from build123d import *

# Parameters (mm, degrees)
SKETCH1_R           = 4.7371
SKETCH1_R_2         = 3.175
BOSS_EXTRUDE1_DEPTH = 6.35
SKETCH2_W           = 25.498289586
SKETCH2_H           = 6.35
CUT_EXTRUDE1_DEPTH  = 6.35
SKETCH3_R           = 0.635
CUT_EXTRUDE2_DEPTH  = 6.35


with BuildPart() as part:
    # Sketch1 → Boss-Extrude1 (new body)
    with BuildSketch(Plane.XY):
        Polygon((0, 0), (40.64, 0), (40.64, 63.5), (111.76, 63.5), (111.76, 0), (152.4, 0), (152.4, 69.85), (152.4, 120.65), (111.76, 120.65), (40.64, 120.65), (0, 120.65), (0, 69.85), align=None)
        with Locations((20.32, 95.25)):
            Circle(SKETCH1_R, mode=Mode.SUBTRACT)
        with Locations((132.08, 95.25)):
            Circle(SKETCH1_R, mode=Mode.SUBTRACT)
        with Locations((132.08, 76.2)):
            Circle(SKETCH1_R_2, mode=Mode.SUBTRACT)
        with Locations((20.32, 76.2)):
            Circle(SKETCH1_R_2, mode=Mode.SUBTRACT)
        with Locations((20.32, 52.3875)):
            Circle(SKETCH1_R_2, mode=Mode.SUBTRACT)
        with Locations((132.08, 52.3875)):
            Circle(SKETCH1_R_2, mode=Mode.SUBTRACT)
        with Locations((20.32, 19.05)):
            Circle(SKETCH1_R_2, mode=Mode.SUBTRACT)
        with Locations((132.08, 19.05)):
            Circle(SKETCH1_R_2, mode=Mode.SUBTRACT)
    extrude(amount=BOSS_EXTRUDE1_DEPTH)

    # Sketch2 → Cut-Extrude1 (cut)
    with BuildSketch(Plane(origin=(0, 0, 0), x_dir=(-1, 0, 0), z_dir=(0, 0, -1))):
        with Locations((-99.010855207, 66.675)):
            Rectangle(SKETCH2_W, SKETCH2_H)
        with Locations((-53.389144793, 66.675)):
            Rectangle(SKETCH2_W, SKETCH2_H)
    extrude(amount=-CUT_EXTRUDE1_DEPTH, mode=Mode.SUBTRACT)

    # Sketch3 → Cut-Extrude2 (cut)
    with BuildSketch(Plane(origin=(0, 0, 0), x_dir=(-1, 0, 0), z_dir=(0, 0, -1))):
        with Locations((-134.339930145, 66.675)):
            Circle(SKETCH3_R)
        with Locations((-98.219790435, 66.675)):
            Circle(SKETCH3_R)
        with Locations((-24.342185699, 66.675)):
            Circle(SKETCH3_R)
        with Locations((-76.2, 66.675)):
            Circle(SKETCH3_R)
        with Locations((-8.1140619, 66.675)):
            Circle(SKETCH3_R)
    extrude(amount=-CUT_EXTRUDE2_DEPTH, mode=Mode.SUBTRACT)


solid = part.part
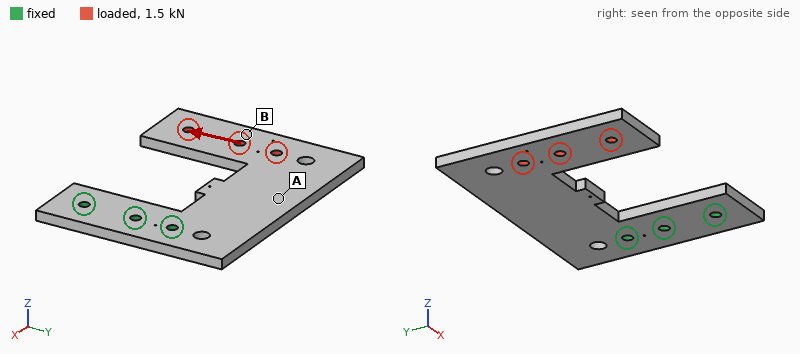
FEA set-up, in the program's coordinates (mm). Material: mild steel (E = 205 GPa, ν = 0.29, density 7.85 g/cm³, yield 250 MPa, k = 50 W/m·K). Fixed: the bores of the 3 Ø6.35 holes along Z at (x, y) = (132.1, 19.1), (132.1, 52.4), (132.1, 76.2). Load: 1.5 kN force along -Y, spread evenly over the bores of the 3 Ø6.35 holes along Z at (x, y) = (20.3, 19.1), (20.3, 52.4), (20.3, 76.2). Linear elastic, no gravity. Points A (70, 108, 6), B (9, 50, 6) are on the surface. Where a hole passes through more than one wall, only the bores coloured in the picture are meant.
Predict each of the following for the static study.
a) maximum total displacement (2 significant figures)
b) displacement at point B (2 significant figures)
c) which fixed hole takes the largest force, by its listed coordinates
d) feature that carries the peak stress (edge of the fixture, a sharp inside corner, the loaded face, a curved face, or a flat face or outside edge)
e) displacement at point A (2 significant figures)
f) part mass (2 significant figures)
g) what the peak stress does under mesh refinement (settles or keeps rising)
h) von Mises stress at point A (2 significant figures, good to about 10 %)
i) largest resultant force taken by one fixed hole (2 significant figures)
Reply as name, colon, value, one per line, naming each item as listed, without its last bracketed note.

maximum total displacement: 0.18 mm
displacement at point B: 0.14 mm
which fixed hole takes the largest force, by its listed coordinates: (132.1, 76.2)
feature that carries the peak stress: edge of the fixture
displacement at point A: 0.063 mm
part mass: 660 g
what the peak stress does under mesh refinement: keeps rising
von Mises stress at point A: 16 MPa
largest resultant force taken by one fixed hole: 4.4 kN
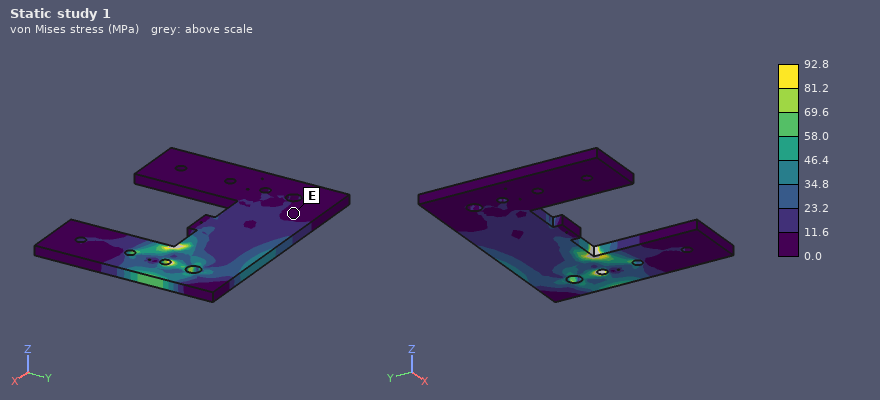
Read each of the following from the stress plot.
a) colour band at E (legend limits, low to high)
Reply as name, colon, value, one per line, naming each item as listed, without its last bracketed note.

colour band at E: 0.0 to 11.6 MPa
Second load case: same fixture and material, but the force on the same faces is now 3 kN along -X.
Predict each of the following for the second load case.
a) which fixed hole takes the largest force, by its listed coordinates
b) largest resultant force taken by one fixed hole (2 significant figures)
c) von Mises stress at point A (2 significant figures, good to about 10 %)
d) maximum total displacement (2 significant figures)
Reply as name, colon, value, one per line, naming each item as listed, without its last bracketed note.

which fixed hole takes the largest force, by its listed coordinates: (132.1, 52.4)
largest resultant force taken by one fixed hole: 2.1 kN
von Mises stress at point A: 15 MPa
maximum total displacement: 0.19 mm
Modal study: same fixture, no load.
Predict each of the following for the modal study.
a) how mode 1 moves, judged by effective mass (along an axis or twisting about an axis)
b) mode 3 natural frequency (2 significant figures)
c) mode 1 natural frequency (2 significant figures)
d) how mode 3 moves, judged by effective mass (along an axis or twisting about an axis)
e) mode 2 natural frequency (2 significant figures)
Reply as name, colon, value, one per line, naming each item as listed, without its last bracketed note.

how mode 1 moves, judged by effective mass: along Z
mode 3 natural frequency: 970 Hz
mode 1 natural frequency: 190 Hz
how mode 3 moves, judged by effective mass: along Y
mode 2 natural frequency: 430 Hz
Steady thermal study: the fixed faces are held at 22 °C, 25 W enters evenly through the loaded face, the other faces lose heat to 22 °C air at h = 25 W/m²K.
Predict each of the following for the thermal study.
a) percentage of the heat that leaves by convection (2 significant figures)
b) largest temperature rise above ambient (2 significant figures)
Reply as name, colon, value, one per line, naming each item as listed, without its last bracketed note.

percentage of the heat that leaves by convection: 84 %
largest temperature rise above ambient: 75 K
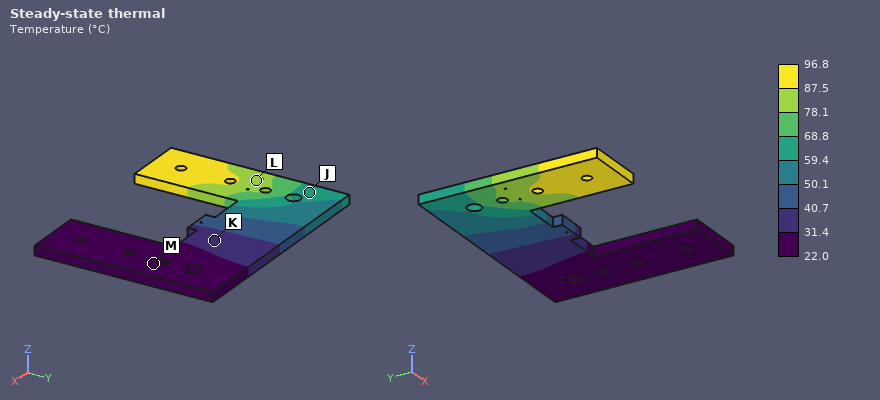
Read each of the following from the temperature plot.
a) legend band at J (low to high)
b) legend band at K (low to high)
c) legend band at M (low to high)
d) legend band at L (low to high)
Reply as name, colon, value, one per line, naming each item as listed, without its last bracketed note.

legend band at J: 59.4 to 68.8 °C
legend band at K: 31.4 to 40.7 °C
legend band at M: 22.0 to 31.4 °C
legend band at L: 78.1 to 87.5 °C
